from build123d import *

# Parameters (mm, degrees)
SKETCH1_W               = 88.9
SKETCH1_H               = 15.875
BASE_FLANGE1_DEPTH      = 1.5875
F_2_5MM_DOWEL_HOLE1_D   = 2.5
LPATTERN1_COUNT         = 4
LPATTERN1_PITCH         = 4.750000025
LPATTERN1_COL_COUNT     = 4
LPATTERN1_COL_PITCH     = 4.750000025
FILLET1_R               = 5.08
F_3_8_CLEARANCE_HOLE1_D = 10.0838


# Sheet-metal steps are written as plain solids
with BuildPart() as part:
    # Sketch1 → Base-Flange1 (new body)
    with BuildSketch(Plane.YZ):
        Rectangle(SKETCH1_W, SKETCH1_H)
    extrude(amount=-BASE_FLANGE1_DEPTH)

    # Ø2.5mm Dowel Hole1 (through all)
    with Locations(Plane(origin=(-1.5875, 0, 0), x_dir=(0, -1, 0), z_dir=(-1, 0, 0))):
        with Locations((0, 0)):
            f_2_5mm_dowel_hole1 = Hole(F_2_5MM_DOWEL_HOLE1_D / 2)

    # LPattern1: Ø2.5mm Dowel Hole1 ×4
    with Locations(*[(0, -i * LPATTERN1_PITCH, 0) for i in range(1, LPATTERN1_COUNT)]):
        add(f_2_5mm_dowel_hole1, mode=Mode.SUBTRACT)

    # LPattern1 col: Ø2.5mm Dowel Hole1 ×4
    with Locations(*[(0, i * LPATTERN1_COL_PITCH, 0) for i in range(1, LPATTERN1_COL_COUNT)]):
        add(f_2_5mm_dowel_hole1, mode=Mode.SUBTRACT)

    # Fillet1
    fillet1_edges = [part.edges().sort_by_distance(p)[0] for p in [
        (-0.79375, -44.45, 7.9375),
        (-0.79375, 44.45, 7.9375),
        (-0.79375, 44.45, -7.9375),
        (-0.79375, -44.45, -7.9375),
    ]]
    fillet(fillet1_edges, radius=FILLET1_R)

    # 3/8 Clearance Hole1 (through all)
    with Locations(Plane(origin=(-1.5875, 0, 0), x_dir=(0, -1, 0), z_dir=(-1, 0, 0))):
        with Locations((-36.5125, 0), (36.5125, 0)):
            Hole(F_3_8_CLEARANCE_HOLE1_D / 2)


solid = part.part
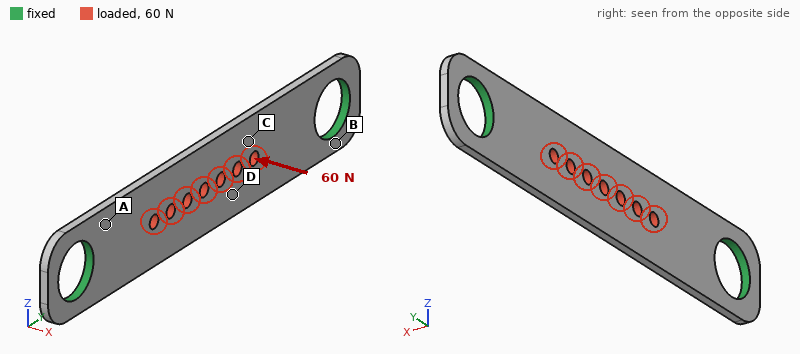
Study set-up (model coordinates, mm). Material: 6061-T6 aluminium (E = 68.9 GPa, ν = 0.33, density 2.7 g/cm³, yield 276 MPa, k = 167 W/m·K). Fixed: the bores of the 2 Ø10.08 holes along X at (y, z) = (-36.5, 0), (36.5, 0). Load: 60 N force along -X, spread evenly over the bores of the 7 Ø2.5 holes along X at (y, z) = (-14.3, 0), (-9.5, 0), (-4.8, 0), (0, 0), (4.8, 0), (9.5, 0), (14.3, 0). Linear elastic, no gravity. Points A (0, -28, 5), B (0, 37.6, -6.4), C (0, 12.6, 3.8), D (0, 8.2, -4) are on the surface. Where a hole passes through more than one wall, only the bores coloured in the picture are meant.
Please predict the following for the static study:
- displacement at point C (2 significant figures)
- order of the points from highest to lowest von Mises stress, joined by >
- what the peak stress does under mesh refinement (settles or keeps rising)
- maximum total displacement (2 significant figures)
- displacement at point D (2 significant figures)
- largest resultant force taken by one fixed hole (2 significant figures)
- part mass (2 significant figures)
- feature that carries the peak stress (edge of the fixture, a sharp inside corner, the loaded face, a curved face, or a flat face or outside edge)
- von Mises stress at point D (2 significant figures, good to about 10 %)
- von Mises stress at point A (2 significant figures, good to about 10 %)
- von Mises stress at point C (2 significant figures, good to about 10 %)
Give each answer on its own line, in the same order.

0.13 mm
A > D > C > B
keeps rising
0.19 mm
0.16 mm
30 N
5.1 g
edge of the fixture
32 MPa
45 MPa
19 MPa
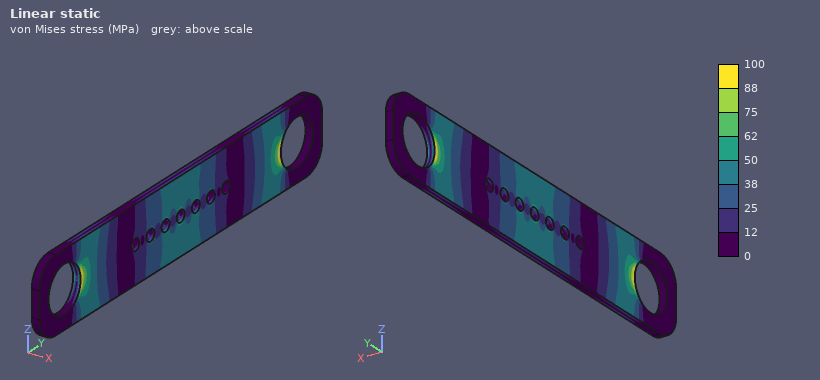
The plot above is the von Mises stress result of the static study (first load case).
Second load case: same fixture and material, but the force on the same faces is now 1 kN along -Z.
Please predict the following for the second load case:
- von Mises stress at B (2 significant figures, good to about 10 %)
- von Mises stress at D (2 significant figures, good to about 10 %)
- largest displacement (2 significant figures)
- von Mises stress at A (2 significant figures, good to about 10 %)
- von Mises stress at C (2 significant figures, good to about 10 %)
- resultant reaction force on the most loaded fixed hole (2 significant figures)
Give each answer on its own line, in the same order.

29 MPa
39 MPa
68 µm
52 MPa
40 MPa
500 N
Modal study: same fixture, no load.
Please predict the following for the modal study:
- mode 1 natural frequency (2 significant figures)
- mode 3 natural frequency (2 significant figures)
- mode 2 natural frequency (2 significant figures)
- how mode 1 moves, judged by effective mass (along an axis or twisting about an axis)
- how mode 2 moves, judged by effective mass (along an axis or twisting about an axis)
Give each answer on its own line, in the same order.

2000 Hz
5400 Hz
5000 Hz
along X
twisting about Y
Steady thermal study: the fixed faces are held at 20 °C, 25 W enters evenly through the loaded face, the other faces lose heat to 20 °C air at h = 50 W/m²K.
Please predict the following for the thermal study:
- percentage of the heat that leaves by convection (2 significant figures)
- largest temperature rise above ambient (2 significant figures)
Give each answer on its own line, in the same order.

17 %
68 K
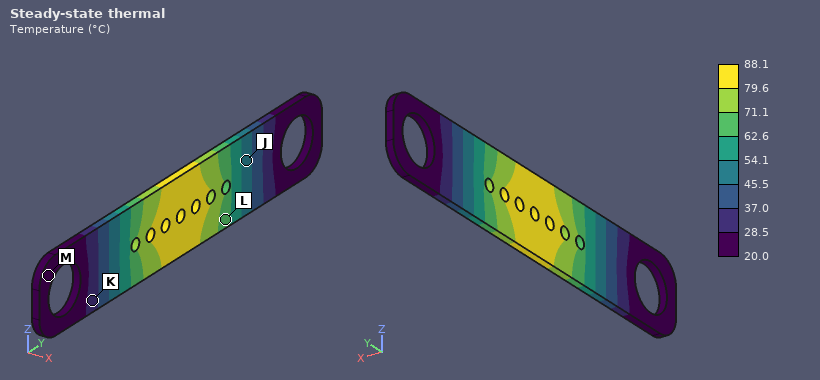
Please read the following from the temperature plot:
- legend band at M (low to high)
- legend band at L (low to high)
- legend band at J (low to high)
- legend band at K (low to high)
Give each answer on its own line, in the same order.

20.0 to 28.5 °C
62.6 to 71.1 °C
45.5 to 54.1 °C
28.5 to 37.0 °C
